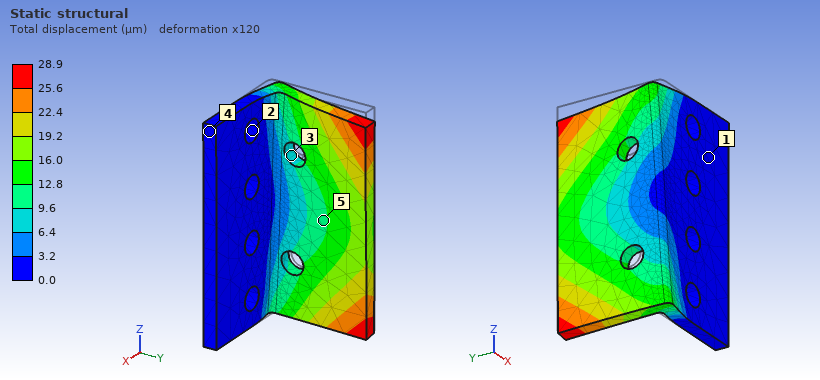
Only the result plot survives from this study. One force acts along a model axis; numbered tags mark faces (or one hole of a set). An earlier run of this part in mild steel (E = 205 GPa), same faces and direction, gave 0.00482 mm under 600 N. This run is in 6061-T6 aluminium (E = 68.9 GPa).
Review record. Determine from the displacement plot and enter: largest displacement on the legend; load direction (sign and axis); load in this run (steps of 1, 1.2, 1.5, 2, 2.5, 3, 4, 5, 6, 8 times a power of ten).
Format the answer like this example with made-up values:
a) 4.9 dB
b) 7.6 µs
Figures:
a) 28.9 µm
b) -Z
c) 1.2 kN
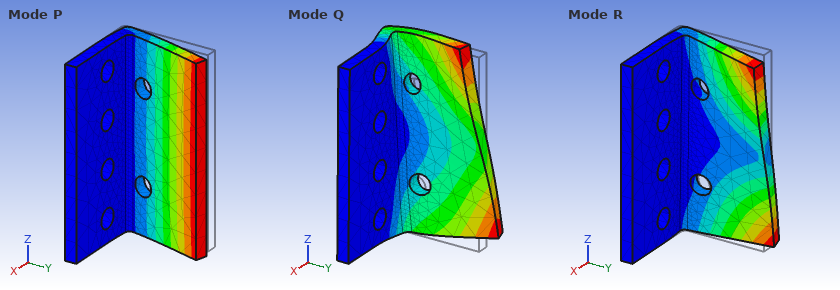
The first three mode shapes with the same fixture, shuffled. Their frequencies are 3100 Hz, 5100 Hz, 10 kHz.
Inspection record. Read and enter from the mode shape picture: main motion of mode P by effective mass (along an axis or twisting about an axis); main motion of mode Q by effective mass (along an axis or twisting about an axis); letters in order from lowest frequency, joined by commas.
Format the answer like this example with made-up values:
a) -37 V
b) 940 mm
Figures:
a) along X
b) along Z
c) P, R, Q
